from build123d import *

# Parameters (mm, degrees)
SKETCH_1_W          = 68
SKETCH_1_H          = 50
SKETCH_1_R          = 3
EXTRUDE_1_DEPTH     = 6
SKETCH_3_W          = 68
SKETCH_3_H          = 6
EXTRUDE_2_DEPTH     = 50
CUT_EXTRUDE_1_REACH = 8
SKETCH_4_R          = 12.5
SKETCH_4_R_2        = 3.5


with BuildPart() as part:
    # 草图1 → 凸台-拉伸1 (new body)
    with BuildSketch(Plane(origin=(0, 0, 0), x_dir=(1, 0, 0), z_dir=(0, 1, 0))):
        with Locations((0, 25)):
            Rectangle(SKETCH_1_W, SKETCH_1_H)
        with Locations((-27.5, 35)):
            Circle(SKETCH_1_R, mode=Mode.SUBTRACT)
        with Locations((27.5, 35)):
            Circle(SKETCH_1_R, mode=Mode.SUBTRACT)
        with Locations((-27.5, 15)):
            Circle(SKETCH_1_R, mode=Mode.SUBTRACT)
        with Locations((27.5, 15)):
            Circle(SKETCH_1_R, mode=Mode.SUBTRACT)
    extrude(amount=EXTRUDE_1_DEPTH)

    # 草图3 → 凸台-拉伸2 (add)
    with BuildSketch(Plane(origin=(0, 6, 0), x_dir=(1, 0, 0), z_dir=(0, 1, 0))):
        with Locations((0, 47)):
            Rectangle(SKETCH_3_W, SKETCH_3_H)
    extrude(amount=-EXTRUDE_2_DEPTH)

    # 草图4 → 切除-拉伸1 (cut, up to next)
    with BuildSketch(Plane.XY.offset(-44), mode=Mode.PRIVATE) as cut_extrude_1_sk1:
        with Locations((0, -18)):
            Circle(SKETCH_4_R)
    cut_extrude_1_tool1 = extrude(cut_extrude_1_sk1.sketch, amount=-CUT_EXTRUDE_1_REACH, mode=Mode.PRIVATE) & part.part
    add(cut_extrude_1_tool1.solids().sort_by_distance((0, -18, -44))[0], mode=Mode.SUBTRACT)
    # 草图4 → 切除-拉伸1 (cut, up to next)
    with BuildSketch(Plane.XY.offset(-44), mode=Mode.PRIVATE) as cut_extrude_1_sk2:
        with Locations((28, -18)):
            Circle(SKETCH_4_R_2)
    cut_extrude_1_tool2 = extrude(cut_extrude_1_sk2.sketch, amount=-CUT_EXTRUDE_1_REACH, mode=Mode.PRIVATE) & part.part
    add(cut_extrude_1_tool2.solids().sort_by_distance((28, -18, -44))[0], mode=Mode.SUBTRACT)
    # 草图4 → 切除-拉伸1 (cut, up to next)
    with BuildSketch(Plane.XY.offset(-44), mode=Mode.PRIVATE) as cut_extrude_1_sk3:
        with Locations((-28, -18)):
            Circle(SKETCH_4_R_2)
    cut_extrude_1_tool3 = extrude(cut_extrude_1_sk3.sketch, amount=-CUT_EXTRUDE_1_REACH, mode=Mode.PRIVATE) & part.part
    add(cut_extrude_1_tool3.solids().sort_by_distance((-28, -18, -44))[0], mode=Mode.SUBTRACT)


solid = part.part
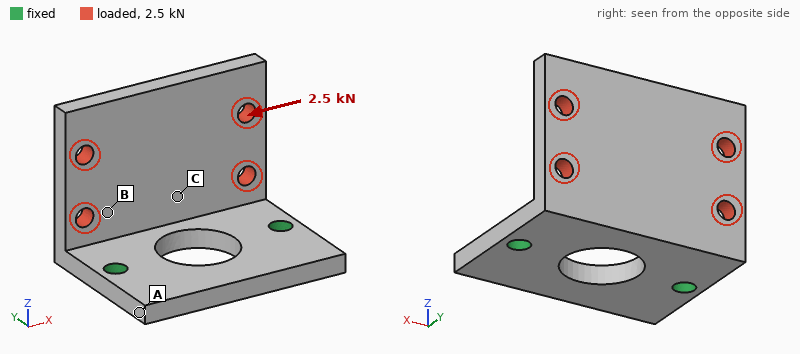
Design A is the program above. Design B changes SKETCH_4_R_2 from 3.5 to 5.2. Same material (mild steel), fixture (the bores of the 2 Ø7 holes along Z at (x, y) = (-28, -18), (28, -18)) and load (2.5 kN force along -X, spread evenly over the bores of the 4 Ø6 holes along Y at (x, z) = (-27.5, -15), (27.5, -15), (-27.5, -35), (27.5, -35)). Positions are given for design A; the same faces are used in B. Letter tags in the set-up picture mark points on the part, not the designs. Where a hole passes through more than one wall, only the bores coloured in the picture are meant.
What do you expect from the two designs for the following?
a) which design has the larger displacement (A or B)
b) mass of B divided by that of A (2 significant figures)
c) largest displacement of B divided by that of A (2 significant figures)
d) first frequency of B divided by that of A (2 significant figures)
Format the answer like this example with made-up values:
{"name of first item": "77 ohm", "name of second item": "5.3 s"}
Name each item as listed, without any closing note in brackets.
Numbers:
{"which design has the larger displacement": "A", "mass of B divided by that of A": "0.98", "largest displacement of B divided by that of A": "0.81", "first frequency of B divided by that of A": "1.1"}
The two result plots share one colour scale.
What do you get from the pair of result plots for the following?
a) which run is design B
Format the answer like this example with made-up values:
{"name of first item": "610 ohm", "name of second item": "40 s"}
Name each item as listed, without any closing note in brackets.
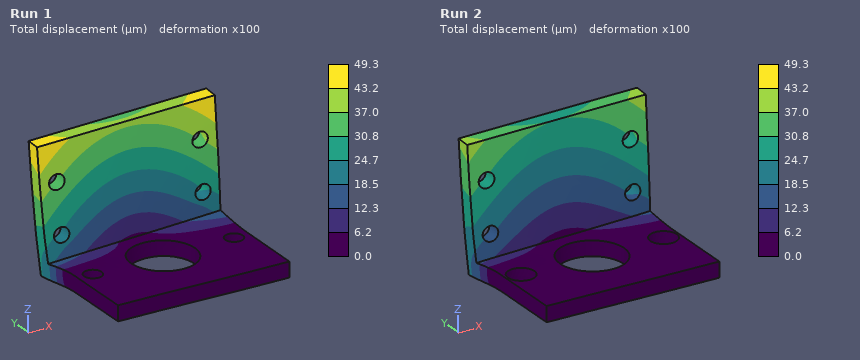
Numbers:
{"which run is design B": "Run 2"}
